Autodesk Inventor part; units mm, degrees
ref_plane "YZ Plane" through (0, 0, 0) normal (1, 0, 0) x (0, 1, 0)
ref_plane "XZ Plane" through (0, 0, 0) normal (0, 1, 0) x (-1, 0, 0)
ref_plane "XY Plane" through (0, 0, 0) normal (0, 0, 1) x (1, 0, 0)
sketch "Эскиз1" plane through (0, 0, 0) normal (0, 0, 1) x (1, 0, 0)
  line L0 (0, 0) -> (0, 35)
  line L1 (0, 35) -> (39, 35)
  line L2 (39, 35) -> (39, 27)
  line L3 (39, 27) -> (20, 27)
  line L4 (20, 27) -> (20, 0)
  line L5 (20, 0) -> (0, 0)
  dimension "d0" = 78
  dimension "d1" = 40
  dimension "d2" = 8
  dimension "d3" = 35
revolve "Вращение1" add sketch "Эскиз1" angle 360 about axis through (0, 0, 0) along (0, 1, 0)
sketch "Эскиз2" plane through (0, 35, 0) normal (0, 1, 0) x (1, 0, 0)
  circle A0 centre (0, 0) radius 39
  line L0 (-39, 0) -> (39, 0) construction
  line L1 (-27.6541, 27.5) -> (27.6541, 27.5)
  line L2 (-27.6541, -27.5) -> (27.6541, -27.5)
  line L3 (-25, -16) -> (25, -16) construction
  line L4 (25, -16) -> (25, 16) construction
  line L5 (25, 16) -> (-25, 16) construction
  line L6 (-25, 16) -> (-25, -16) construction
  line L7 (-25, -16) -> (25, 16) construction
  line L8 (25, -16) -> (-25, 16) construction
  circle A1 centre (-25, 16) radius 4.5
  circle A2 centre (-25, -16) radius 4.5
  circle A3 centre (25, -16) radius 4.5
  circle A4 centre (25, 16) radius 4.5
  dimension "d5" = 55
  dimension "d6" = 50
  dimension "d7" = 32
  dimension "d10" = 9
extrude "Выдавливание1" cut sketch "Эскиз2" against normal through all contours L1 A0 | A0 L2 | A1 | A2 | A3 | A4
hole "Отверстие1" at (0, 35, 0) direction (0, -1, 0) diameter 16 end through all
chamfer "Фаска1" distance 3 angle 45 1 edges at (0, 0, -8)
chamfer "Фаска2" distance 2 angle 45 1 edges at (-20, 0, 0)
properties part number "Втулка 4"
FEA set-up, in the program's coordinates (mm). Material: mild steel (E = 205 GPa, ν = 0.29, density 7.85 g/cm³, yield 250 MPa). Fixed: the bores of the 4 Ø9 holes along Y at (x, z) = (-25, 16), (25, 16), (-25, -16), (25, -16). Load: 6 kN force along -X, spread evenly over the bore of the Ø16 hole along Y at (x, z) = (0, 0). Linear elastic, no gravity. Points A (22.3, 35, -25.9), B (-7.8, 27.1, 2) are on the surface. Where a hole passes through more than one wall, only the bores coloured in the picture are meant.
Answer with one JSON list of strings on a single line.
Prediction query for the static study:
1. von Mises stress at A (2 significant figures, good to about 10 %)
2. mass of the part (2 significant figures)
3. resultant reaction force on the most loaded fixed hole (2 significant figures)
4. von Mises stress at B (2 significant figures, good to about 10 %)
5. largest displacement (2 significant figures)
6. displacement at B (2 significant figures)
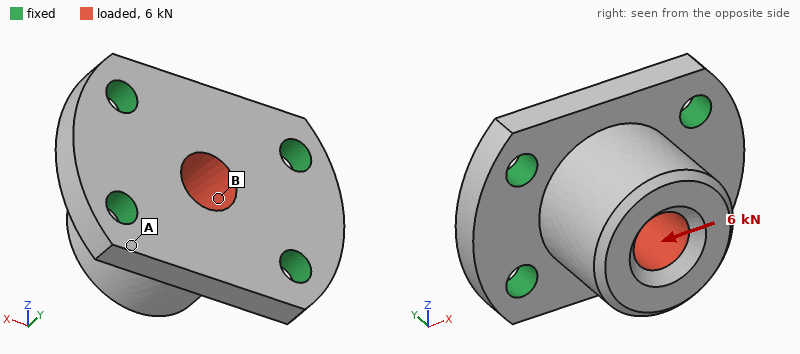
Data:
["3.1 MPa", "440 g", "1.8 kN", "7.1 MPa", "3.8 µm", "1.0 µm"]
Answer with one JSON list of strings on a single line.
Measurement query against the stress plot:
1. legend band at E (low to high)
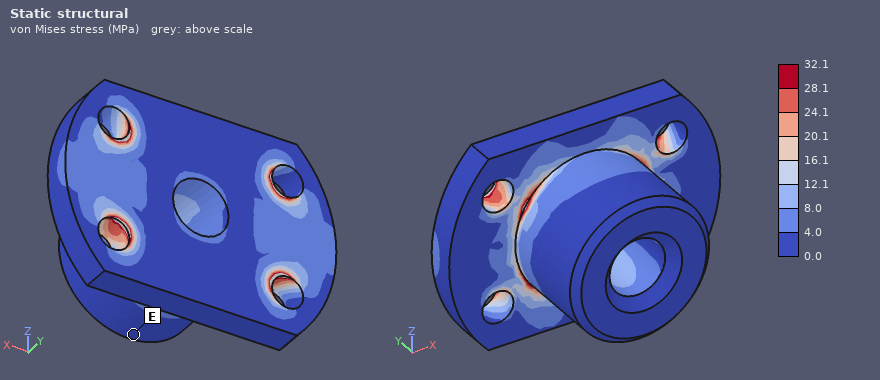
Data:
["0.0 to 4.0 MPa"]
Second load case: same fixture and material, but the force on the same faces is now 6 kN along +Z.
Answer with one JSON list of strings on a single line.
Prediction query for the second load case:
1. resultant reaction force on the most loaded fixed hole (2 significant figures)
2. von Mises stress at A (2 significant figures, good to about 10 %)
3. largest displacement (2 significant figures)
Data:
["2.0 kN", "12 MPa", "6.6 µm"]
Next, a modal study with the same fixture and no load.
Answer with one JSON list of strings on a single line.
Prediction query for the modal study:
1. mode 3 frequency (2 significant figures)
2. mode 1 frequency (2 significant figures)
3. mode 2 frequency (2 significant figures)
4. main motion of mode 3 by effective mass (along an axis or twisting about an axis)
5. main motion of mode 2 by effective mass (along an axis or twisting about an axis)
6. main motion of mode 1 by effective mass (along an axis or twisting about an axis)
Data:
["14 kHz", "9400 Hz", "13 kHz", "along Y", "along X", "along Z"]
